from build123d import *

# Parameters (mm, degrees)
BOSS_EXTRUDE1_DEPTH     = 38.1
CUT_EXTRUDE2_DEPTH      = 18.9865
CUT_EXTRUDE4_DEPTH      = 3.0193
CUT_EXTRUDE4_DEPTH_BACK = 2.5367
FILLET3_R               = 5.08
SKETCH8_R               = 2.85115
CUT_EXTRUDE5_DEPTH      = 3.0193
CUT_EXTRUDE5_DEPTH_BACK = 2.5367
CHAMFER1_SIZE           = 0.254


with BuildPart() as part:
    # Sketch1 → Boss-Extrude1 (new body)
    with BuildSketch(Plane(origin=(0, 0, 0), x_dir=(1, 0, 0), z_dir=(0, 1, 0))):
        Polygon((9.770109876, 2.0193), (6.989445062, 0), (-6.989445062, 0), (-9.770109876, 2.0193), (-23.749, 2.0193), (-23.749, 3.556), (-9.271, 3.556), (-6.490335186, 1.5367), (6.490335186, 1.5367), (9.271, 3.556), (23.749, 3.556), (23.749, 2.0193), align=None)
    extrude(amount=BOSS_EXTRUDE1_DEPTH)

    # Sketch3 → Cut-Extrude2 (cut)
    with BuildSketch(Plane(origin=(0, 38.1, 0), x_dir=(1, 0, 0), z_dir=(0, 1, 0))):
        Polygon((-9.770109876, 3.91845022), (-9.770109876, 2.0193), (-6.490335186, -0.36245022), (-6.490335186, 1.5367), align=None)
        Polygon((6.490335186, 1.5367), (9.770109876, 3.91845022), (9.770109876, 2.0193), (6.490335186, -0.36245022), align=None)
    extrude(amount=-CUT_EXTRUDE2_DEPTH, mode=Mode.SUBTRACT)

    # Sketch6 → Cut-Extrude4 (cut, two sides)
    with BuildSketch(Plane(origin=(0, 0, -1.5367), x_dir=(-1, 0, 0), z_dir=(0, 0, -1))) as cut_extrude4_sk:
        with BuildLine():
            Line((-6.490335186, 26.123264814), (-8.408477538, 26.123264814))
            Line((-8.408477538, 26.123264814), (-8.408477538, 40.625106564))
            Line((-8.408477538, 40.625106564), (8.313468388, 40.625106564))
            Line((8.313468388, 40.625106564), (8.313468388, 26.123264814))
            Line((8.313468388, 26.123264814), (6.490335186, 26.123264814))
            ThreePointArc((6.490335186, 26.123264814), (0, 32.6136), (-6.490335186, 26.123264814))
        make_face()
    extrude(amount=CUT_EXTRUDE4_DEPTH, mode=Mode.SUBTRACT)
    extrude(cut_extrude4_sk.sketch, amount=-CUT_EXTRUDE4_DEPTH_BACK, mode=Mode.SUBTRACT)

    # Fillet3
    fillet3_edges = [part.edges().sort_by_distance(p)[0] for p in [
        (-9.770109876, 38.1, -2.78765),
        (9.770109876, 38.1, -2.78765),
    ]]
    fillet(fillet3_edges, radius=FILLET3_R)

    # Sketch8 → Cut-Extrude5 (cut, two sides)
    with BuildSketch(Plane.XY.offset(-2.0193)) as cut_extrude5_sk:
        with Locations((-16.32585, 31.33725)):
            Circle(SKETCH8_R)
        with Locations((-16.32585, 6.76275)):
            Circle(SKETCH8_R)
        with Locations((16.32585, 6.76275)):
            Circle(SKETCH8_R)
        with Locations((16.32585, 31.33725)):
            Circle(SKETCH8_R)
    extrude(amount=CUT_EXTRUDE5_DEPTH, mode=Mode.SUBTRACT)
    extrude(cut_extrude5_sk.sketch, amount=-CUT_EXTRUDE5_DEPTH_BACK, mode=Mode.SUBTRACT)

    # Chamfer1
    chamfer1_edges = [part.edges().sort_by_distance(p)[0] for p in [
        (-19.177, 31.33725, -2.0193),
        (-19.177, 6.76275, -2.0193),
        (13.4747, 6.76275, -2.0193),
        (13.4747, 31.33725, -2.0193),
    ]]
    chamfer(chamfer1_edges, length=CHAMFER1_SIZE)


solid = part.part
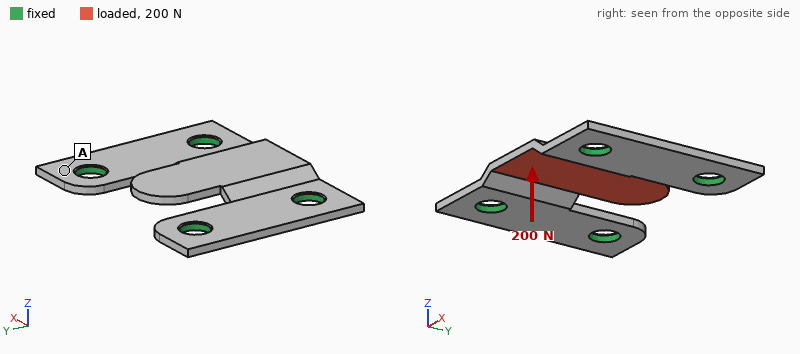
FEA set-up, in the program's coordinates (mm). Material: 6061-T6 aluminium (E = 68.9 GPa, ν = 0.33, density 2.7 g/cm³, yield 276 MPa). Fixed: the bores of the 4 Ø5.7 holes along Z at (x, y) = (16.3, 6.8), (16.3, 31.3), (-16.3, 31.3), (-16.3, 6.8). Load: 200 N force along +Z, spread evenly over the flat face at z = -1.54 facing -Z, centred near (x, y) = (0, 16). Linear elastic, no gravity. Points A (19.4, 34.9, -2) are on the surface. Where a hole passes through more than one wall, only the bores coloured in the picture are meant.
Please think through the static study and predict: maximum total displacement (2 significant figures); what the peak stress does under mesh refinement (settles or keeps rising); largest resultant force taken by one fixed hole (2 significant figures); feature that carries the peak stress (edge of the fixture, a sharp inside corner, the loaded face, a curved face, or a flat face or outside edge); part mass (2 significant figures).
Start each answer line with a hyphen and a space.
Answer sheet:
- 0.29 mm
- keeps rising
- 240 N
- a sharp inside corner
- 6.2 g
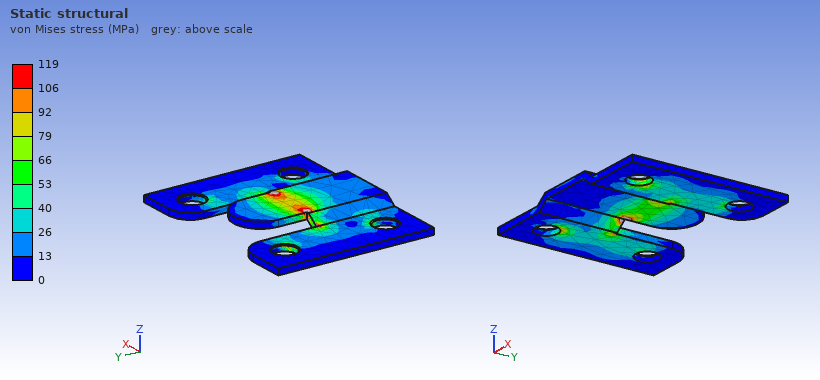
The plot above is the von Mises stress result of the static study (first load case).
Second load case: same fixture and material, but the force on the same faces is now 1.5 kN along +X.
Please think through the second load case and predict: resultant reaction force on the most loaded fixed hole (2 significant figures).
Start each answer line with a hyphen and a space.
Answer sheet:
- 730 N
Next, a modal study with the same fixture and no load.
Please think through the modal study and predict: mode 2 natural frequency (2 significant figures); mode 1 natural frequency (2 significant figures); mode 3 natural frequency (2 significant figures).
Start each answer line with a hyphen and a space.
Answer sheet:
- 13 kHz
- 4100 Hz
- 13 kHz
